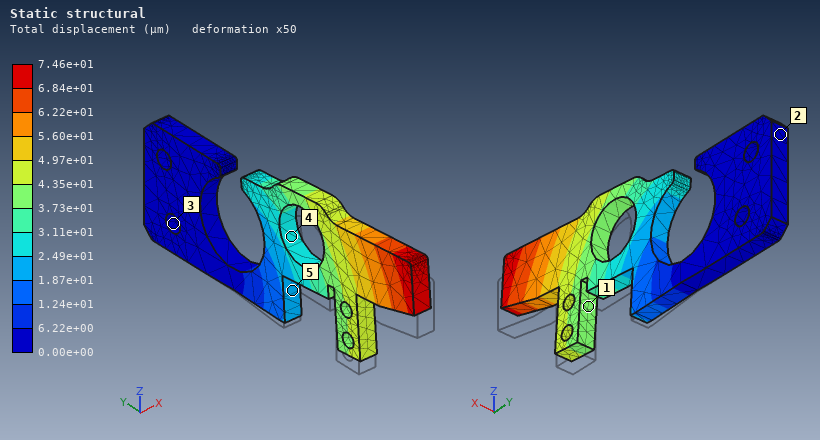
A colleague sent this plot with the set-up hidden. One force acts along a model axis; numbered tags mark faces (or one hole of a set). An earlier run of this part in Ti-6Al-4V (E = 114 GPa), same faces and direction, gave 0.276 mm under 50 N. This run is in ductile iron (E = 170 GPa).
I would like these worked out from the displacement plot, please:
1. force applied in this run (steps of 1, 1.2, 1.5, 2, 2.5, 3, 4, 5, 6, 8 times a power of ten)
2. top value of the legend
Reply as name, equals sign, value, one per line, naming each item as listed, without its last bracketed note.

force applied in this run = 20 N
top value of the legend = 7.46e+01 µm
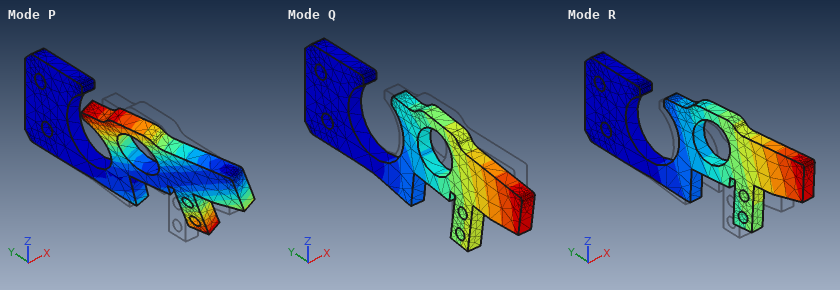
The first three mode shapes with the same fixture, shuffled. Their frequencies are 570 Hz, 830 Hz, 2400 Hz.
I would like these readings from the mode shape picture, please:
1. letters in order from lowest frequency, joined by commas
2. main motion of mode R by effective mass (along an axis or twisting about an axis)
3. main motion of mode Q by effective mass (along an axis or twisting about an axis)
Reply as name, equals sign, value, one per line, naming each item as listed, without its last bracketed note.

letters in order from lowest frequency, joined by commas = R, Q, P
main motion of mode R by effective mass = along X
main motion of mode Q by effective mass = along Z
